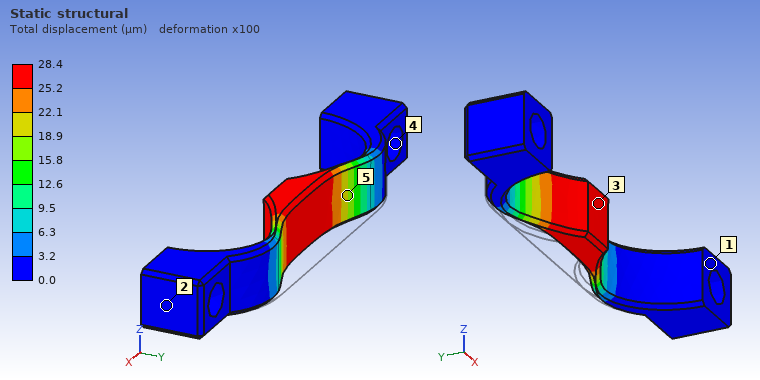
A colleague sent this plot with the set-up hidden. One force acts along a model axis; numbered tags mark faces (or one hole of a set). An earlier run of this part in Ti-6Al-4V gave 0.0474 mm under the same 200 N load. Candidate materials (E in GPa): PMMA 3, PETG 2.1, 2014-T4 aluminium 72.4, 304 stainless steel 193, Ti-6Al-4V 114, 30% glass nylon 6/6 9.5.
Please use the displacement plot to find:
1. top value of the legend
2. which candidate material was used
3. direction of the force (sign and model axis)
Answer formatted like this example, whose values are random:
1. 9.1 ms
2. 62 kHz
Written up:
1. 28.4 µm
2. 304 stainless steel
3. -Y
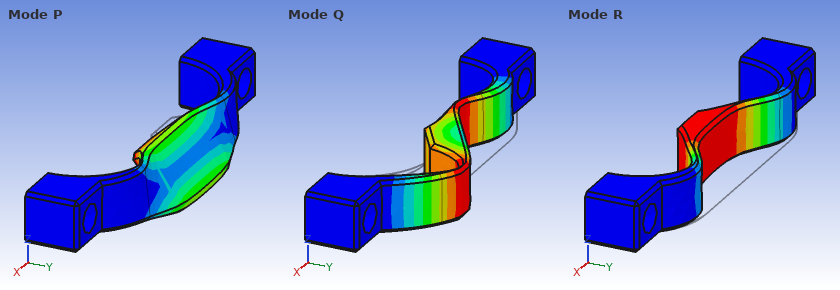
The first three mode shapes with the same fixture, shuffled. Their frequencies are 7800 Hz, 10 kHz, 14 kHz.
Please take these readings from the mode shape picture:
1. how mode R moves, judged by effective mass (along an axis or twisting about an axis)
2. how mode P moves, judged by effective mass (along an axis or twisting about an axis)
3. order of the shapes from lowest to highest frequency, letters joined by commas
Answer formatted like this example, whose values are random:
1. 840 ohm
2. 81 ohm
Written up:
1. along Y
2. along Z
3. R, P, Q
